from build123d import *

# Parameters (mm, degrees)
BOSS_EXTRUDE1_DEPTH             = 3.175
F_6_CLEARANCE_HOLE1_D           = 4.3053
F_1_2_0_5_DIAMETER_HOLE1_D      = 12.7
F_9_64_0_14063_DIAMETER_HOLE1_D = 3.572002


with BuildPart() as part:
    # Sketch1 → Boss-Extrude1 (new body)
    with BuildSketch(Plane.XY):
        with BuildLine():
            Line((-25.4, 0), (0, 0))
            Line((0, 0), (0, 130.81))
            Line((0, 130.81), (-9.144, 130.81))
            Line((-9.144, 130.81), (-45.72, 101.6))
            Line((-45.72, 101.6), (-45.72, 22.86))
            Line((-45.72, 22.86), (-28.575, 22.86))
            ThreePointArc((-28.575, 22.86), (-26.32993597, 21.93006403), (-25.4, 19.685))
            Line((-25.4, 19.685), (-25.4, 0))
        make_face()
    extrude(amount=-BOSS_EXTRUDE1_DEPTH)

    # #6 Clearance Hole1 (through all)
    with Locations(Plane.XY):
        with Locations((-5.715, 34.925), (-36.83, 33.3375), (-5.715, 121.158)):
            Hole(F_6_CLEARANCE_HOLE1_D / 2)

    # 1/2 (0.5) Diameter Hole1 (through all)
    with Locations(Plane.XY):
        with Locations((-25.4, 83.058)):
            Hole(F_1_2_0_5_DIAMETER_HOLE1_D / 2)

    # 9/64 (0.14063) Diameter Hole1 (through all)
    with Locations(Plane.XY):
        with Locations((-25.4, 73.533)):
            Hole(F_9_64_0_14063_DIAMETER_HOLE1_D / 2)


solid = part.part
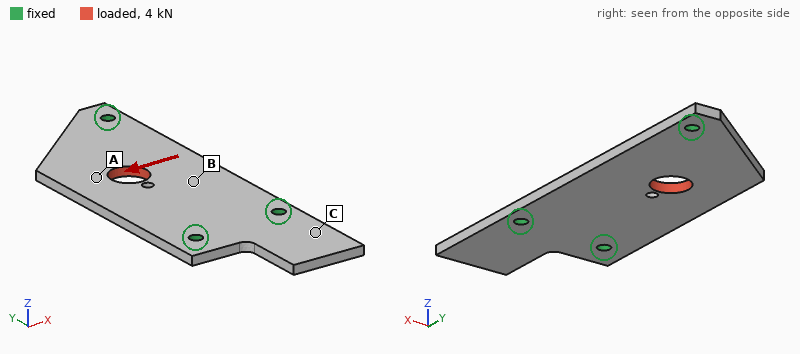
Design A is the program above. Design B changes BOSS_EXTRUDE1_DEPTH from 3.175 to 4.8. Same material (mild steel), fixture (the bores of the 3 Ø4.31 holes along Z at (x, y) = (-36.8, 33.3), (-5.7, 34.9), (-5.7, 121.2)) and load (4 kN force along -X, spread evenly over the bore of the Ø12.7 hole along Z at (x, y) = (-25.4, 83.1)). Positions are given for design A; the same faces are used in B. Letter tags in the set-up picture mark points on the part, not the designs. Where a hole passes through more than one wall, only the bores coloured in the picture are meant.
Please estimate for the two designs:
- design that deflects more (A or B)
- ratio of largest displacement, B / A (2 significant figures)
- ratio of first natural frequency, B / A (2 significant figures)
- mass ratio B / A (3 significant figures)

A
0.66
1.5
1.51
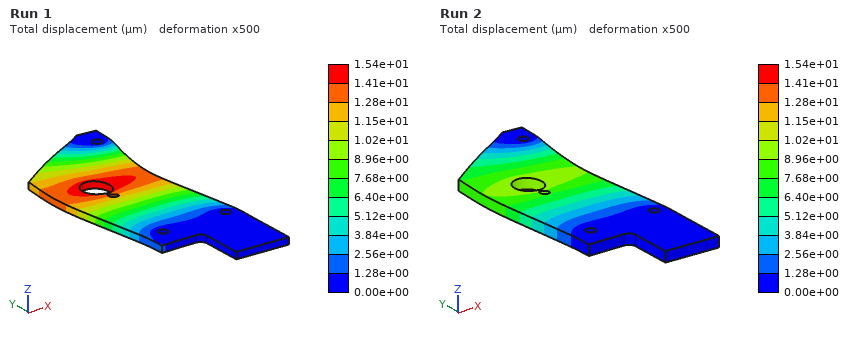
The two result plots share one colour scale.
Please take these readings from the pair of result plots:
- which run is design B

Run 2
